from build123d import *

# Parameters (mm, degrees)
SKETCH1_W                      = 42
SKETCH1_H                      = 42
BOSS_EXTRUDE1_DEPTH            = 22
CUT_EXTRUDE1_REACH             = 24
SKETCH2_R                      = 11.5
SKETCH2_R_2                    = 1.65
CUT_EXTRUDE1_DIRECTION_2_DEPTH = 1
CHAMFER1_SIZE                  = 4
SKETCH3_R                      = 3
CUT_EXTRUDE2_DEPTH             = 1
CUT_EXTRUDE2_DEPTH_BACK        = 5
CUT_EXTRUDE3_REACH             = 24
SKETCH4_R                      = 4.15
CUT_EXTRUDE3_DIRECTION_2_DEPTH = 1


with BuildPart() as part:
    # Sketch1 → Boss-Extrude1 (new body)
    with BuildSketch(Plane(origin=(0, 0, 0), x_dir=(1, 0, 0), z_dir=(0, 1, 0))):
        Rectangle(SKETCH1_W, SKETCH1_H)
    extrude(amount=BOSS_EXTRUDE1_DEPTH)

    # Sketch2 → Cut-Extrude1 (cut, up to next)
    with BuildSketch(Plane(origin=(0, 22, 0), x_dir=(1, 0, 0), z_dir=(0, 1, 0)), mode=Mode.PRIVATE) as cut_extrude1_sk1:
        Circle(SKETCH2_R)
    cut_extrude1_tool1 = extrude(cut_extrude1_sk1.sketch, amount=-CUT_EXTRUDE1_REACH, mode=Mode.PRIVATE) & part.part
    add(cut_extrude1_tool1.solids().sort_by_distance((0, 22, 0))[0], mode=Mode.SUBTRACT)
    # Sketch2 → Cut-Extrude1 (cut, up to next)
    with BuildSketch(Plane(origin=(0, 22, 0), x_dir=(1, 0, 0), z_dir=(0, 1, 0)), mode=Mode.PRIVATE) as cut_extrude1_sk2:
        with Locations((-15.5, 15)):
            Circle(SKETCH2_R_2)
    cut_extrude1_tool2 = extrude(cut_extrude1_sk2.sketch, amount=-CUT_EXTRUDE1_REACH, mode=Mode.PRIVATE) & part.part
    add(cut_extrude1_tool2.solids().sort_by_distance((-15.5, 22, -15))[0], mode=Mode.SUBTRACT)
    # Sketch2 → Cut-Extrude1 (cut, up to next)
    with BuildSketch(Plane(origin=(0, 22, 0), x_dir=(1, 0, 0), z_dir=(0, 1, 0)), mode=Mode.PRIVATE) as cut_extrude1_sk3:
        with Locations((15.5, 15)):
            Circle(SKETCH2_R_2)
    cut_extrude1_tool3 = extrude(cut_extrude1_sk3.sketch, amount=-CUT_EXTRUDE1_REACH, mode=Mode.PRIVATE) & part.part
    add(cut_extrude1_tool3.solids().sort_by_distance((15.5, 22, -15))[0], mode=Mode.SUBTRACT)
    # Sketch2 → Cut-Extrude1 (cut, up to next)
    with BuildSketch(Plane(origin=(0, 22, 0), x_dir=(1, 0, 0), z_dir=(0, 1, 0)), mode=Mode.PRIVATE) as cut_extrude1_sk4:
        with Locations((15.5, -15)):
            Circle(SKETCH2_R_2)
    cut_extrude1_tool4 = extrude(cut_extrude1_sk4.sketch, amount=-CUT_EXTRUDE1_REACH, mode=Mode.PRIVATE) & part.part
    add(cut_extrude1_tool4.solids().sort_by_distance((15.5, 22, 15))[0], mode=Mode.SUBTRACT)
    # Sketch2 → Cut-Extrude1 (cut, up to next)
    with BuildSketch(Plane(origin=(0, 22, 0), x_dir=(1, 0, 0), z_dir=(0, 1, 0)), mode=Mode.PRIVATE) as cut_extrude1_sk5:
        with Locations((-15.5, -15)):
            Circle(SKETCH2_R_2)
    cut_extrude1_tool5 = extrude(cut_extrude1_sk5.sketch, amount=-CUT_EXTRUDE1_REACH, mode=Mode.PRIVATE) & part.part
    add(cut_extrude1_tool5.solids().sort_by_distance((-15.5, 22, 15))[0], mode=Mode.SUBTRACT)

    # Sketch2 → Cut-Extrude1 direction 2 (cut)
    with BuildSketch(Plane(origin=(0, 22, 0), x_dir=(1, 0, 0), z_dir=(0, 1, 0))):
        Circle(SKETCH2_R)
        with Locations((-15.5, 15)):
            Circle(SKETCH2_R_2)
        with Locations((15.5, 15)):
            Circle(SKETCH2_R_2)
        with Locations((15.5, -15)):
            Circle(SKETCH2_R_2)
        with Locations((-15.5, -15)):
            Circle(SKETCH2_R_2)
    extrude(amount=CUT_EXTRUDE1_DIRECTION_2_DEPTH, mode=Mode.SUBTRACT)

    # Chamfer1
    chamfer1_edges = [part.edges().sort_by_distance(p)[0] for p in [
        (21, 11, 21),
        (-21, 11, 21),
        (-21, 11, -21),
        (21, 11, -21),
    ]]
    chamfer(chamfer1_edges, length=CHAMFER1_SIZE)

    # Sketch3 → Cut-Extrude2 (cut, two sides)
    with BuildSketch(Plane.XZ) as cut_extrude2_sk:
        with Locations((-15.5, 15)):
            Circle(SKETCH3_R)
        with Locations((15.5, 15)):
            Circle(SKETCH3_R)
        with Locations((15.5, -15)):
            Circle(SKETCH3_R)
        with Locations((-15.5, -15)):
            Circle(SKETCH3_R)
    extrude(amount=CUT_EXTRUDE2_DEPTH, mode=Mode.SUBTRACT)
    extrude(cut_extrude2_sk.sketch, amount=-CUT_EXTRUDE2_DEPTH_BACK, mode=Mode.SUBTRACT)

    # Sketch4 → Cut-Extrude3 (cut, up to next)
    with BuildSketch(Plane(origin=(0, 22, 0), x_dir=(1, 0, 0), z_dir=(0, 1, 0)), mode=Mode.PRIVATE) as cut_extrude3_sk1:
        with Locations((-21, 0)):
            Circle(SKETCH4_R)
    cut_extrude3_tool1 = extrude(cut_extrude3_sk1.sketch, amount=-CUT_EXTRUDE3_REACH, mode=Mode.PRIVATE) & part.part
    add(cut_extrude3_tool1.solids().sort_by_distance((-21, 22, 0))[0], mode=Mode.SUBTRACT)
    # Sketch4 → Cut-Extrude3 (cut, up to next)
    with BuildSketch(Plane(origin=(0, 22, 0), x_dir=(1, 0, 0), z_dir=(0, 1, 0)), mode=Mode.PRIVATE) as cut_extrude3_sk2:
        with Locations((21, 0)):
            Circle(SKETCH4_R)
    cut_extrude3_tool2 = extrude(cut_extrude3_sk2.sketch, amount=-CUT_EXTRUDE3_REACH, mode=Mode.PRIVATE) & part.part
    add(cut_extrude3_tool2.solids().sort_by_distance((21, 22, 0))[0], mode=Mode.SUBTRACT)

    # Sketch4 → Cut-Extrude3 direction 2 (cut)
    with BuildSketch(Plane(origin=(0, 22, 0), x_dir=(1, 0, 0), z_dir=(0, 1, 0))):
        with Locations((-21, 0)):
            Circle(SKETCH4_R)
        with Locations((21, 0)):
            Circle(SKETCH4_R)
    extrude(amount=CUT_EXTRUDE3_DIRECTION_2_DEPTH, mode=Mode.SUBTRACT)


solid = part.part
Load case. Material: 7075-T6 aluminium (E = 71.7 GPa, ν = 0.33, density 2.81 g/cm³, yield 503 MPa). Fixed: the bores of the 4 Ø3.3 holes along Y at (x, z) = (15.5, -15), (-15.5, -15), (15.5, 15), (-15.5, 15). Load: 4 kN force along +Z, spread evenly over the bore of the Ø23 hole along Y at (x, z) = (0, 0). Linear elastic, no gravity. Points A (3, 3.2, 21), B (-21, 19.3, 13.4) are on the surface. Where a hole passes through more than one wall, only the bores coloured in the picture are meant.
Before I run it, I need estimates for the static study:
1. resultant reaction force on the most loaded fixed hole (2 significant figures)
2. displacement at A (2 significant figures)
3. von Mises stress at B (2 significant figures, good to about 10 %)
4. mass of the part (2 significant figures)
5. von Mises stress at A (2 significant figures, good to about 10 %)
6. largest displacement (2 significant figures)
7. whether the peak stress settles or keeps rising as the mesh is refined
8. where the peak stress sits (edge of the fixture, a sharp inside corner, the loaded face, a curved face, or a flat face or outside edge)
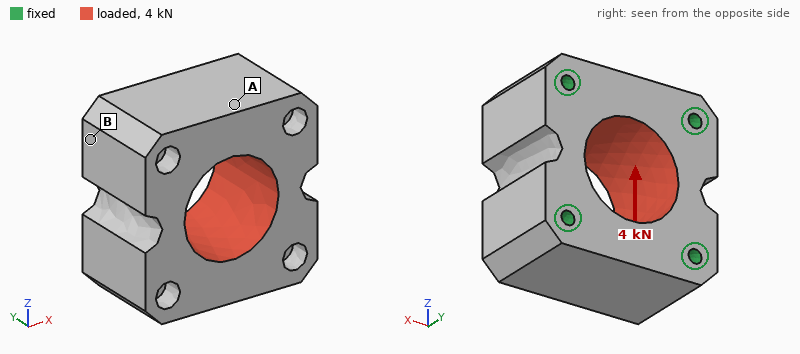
1.0 kN
1.8 µm
1.4 MPa
75 g
5.0 MPa
2.3 µm
keeps rising
edge of the fixture
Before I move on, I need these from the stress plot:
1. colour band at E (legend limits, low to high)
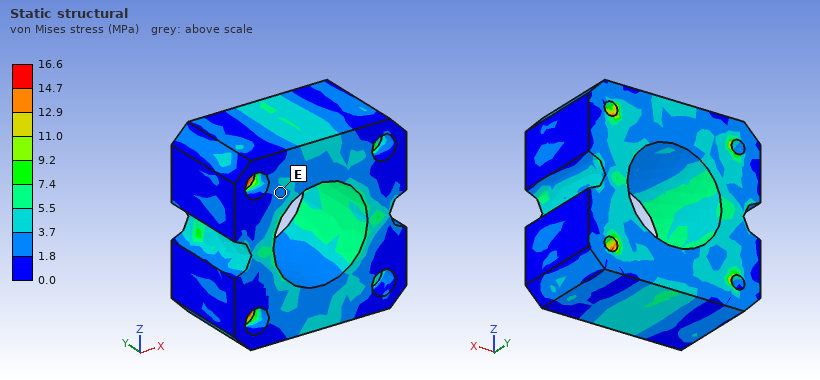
1.8 to 3.7 MPa
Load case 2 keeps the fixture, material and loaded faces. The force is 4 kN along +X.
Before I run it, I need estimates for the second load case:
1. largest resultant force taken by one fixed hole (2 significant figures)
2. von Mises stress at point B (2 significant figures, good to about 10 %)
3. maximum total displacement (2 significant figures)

1.1 kN
3.8 MPa
2.5 µm
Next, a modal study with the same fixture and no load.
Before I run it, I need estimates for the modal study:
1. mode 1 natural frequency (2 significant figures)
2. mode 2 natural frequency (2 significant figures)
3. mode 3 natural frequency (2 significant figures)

25 kHz
37 kHz
38 kHz
